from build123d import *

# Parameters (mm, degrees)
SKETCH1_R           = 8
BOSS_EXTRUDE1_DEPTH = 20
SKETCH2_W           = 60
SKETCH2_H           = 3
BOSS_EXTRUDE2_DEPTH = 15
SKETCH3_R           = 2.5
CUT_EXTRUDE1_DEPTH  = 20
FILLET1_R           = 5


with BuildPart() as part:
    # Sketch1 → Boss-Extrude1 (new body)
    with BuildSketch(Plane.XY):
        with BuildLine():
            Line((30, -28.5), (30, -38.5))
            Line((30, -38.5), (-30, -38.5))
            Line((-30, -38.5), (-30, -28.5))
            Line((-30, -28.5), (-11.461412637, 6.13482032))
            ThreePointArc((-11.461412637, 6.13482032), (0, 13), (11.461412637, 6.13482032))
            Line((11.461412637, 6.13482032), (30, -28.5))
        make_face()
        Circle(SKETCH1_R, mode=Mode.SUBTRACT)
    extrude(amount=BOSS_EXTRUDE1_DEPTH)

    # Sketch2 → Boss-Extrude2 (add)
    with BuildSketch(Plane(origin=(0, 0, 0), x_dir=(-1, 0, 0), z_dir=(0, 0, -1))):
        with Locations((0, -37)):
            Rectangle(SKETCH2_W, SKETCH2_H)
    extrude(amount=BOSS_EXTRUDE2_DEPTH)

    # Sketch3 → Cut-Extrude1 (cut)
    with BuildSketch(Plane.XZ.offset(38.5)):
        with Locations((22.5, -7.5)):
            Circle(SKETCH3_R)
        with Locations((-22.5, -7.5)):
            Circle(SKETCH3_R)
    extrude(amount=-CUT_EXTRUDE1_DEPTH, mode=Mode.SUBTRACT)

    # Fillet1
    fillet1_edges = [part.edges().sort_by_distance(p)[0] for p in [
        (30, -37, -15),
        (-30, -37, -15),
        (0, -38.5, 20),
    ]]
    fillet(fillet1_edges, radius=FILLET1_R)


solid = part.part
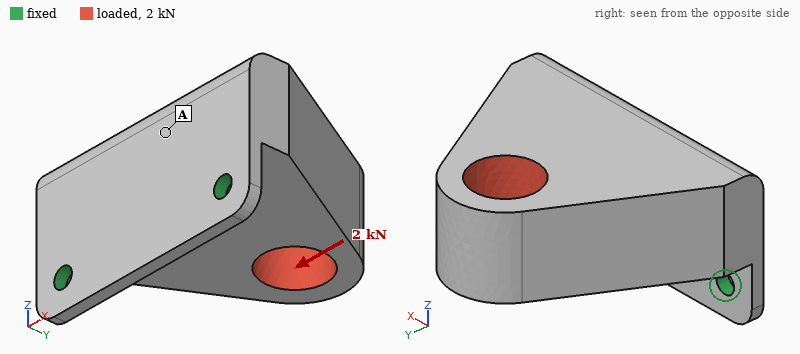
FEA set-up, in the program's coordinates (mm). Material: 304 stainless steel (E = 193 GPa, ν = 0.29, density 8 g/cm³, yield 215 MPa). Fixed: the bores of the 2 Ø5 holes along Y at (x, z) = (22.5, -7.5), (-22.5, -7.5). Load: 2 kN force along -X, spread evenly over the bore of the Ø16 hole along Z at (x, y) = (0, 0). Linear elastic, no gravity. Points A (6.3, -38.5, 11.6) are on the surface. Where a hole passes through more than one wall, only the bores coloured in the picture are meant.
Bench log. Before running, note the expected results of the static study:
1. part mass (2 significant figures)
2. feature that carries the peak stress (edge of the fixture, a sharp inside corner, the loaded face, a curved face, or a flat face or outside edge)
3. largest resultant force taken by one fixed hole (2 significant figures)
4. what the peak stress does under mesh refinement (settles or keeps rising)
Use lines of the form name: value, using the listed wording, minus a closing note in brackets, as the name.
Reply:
part mass: 330 g
feature that carries the peak stress: edge of the fixture
largest resultant force taken by one fixed hole: 2.0 kN
what the peak stress does under mesh refinement: keeps rising
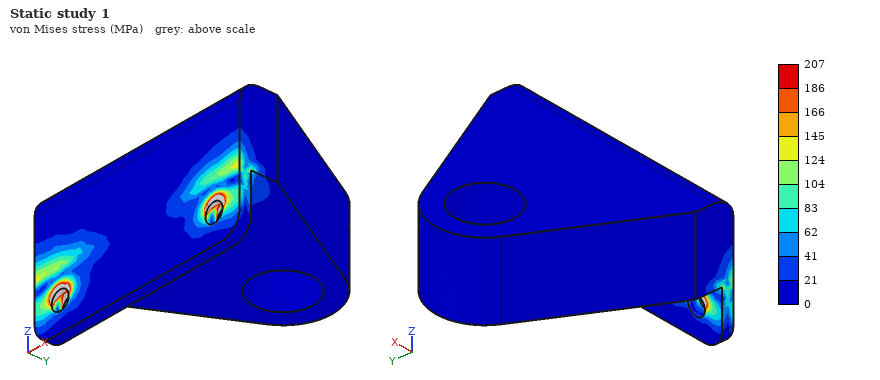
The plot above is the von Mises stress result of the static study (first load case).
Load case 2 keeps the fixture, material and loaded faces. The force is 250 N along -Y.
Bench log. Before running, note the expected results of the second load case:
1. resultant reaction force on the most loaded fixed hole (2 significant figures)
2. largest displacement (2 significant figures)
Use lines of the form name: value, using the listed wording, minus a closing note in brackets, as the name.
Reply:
resultant reaction force on the most loaded fixed hole: 130 N
largest displacement: 68 µm
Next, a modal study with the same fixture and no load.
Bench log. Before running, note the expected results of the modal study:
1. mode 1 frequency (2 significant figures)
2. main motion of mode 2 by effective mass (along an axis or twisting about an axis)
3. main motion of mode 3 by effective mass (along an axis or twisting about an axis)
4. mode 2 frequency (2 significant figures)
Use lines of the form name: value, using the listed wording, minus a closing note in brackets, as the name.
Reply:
mode 1 frequency: 570 Hz
main motion of mode 2 by effective mass: along X
main motion of mode 3 by effective mass: along Y
mode 2 frequency: 3400 Hz
